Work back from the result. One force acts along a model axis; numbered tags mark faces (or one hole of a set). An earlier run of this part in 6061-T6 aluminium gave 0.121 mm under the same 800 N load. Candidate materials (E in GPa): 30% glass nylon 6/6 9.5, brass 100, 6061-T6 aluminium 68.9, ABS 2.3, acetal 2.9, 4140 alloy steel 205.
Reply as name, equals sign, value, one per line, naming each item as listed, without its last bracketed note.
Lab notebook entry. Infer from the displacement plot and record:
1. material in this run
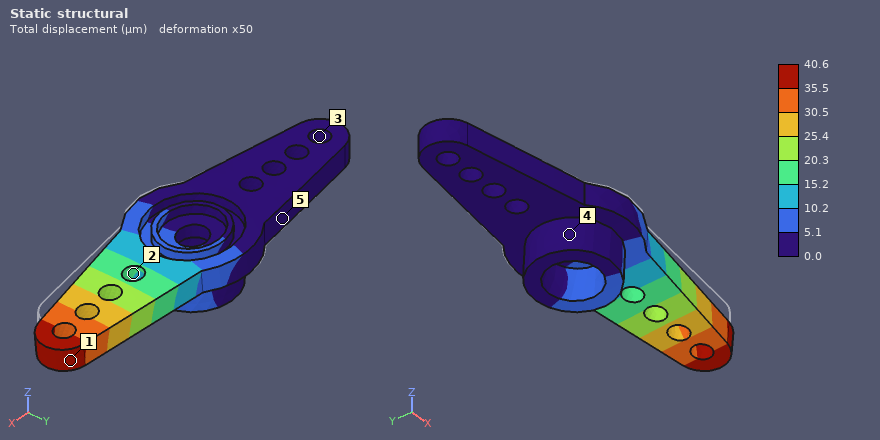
material in this run = 4140 alloy steel
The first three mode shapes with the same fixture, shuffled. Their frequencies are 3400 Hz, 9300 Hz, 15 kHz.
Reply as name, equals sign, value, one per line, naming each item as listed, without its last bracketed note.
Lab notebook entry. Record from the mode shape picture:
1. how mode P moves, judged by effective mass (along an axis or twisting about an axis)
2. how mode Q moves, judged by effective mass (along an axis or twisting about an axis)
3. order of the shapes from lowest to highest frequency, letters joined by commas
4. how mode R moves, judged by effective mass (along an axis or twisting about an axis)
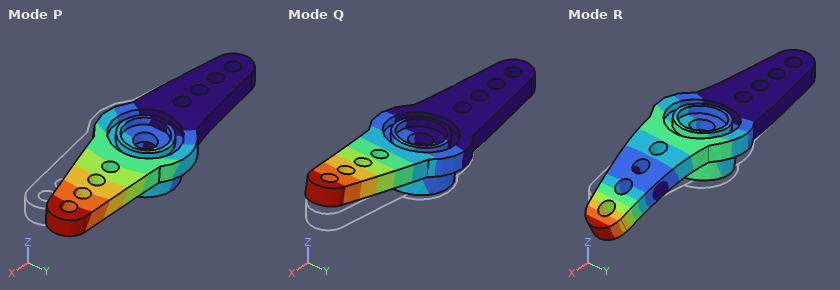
how mode P moves, judged by effective mass = along Y
how mode Q moves, judged by effective mass = along Z
order of the shapes from lowest to highest frequency, letters joined by commas = Q, P, R
how mode R moves, judged by effective mass = along Z
